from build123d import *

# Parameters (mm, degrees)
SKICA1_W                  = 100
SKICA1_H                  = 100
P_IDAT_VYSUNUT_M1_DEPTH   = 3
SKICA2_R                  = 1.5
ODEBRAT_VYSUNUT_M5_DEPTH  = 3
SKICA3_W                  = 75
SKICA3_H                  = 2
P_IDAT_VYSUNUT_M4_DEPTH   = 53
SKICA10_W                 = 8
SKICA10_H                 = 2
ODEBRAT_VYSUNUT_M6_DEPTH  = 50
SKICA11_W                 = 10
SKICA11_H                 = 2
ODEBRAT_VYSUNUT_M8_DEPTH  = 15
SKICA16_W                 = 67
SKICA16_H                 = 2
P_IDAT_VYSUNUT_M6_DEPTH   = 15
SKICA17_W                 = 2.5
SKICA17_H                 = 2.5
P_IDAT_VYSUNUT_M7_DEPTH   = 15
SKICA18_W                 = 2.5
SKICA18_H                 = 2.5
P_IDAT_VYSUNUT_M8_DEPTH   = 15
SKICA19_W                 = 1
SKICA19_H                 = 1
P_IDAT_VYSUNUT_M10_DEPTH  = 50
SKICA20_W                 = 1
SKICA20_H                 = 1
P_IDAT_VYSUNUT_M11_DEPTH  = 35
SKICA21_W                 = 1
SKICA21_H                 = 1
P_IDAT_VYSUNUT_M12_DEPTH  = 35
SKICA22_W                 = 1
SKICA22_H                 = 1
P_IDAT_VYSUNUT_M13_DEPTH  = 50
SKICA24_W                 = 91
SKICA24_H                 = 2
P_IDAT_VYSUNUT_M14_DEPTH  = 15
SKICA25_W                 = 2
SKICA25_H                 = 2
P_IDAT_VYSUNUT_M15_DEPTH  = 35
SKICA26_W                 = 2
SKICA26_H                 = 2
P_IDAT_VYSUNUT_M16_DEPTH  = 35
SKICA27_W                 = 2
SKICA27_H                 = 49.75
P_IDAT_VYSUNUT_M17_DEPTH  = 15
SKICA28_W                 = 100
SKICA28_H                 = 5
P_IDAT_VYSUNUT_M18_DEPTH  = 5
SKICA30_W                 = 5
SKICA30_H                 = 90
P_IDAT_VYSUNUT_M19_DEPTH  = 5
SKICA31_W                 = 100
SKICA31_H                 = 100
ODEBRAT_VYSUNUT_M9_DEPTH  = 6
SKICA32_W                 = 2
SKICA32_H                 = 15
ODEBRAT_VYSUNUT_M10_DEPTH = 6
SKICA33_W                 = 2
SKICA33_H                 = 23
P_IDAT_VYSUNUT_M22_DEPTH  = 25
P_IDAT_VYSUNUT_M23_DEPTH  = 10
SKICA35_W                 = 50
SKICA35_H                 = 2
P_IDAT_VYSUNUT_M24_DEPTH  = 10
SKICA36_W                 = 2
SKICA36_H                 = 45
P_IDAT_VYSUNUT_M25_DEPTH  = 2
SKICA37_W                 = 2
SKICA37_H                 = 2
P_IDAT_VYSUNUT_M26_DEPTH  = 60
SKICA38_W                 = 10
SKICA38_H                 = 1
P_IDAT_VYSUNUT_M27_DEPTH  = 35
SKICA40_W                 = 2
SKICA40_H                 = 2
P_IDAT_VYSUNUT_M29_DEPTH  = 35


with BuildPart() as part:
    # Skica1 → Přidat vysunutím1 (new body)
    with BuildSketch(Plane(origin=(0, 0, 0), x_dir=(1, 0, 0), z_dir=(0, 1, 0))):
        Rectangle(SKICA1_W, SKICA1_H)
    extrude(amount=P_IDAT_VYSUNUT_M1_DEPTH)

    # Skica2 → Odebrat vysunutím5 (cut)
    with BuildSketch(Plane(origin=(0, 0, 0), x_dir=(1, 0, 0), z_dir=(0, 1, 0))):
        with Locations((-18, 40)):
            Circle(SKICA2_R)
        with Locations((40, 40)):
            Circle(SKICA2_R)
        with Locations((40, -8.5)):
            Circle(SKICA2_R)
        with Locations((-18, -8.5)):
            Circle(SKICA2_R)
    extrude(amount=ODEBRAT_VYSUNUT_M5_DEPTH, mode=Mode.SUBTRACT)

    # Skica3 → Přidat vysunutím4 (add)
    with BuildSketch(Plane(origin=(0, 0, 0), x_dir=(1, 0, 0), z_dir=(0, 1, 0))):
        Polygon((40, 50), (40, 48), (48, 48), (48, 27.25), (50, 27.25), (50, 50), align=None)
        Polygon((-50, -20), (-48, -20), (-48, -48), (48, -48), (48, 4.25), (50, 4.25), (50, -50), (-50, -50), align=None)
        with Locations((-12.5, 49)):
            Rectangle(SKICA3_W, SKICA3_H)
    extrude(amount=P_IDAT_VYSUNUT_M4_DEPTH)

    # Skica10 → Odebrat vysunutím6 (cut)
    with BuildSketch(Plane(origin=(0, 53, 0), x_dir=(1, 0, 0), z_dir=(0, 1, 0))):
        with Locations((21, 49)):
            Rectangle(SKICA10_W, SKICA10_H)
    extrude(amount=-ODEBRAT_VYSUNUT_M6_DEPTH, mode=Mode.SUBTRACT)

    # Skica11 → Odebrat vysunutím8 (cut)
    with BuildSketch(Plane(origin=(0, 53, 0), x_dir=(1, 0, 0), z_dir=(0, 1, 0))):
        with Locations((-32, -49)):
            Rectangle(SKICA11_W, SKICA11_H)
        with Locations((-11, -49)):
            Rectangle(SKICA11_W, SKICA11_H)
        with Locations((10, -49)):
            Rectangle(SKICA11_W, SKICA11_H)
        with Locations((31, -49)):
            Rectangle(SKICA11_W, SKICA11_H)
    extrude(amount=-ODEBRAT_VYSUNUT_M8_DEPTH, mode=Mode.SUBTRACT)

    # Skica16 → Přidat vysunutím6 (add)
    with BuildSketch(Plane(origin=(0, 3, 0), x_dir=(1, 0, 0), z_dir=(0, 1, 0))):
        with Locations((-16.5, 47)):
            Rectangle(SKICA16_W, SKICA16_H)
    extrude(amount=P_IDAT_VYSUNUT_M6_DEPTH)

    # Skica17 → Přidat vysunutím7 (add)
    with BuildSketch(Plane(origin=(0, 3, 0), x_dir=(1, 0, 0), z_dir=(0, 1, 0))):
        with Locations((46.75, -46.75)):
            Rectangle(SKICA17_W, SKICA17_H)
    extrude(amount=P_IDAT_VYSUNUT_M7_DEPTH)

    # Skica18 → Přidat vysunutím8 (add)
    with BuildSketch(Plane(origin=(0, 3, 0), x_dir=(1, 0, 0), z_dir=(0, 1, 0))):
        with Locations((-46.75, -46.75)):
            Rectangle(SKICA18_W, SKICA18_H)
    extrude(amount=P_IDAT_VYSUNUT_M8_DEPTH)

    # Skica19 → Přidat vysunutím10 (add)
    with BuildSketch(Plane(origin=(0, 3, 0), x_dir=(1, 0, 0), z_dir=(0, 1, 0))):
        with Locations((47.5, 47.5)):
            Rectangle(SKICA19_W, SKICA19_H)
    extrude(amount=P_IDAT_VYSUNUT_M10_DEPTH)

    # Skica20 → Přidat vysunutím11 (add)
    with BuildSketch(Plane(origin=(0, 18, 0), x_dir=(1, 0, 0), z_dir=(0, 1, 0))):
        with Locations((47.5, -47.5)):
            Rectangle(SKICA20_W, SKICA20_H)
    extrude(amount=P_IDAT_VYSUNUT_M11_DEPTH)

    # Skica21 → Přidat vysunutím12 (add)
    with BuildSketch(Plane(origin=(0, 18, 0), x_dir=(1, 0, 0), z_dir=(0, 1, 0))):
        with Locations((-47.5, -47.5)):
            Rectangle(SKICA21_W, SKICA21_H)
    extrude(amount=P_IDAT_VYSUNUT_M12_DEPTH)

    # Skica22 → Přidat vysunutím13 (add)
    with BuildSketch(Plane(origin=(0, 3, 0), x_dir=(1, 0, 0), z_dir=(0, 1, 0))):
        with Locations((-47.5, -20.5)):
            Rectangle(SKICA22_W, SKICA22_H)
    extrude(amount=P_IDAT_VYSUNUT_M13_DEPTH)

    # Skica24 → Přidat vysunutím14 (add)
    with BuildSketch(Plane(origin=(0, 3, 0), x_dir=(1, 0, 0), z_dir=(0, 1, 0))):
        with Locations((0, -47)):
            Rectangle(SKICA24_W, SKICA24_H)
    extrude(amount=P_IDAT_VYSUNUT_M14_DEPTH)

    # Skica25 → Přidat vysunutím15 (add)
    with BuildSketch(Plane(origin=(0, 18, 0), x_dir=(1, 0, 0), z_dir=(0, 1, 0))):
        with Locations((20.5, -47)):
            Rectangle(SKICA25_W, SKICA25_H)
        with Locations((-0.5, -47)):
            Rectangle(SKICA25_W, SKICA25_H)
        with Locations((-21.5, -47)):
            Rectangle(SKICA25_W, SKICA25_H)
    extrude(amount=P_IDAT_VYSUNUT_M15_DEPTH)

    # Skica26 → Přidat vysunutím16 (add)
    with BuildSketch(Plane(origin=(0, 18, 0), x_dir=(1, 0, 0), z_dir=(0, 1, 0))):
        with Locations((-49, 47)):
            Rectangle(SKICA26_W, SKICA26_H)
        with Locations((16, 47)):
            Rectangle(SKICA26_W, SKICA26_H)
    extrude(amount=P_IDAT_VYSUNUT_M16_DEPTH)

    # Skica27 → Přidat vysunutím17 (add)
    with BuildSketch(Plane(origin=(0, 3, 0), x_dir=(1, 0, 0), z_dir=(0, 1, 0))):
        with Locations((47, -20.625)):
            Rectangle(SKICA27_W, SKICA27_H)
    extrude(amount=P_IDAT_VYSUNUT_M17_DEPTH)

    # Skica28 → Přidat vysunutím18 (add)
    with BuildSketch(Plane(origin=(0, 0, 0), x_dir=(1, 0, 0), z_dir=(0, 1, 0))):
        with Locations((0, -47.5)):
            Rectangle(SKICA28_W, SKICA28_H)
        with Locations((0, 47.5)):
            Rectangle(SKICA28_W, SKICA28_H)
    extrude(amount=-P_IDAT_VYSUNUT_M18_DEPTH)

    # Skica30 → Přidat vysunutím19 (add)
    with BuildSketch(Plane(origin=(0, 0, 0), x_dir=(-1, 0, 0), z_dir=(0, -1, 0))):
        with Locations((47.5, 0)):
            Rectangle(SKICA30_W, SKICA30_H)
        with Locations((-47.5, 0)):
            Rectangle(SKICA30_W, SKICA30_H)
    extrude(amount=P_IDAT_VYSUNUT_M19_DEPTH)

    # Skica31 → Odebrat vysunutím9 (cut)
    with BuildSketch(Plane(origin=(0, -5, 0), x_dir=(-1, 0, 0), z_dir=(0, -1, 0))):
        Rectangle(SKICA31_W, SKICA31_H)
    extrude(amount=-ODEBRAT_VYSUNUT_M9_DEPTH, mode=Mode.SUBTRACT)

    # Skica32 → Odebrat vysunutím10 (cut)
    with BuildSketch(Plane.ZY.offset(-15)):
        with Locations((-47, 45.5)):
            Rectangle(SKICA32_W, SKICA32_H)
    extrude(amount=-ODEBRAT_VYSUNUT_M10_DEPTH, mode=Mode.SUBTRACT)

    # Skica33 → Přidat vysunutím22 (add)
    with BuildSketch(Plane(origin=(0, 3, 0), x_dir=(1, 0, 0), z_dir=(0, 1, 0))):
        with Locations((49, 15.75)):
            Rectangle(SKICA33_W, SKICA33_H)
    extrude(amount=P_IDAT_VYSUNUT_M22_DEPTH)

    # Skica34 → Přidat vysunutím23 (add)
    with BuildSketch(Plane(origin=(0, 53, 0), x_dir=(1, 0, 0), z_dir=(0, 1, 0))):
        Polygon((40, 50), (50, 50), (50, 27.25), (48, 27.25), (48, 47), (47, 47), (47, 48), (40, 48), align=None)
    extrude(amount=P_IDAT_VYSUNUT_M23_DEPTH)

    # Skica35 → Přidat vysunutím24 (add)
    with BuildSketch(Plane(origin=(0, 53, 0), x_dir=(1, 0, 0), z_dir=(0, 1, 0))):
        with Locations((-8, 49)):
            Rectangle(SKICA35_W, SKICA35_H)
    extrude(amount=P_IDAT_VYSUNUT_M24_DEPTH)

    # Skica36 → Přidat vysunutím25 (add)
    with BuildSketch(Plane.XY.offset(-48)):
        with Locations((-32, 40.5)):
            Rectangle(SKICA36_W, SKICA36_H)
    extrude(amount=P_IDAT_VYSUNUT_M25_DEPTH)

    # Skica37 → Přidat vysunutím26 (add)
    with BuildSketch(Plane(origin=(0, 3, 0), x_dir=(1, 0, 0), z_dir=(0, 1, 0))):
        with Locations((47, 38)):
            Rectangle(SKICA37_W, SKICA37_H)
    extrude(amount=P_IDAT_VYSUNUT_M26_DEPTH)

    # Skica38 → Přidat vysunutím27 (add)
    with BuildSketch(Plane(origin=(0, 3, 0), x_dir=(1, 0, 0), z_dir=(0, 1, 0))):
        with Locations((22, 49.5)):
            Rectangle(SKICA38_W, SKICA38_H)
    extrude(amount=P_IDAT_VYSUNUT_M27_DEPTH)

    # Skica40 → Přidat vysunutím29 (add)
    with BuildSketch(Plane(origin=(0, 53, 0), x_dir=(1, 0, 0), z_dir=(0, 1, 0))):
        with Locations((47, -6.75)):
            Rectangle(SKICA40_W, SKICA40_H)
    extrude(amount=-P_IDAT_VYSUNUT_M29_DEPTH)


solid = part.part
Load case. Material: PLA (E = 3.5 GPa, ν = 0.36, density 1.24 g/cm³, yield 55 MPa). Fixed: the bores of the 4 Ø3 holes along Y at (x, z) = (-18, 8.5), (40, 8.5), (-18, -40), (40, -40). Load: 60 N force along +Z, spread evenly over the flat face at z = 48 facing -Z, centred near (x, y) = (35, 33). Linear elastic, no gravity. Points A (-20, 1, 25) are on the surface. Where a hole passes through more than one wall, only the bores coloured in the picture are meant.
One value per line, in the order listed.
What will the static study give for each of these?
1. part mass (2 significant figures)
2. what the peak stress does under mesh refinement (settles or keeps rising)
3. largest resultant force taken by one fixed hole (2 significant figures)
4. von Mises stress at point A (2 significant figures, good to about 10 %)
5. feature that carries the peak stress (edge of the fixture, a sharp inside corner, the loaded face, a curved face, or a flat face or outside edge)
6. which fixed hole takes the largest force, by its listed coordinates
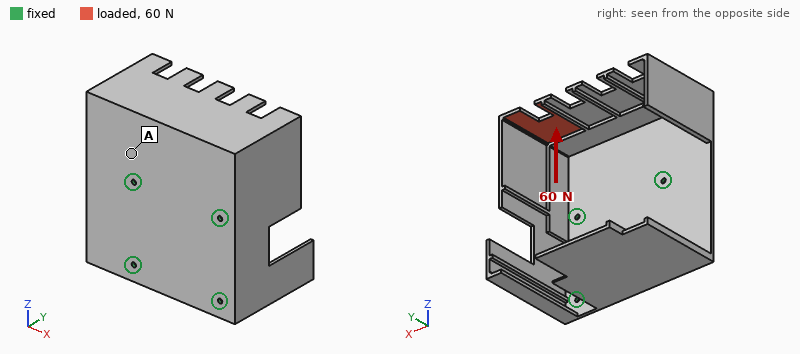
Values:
71 g
keeps rising
53 N
1.3 MPa
edge of the fixture
(40, -40)
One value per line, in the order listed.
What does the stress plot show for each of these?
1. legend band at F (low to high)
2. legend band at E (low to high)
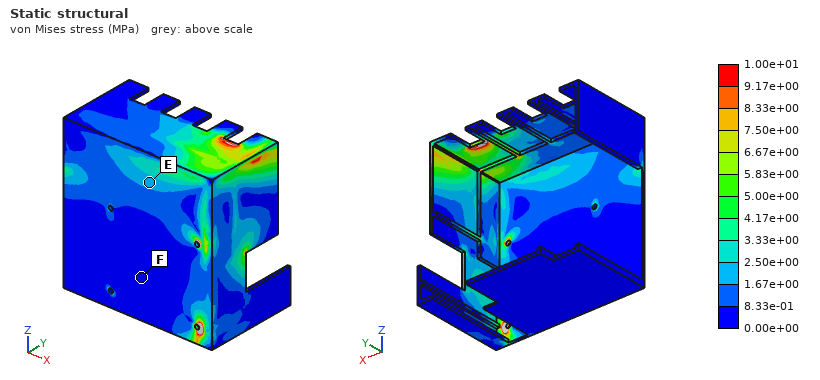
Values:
0.00e+00 to 8.33e-01 MPa
1.67e+00 to 2.50e+00 MPa
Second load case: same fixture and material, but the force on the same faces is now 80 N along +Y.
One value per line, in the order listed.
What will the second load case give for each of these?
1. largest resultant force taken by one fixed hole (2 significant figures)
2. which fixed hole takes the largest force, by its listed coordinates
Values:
140 N
(40, 8.5)
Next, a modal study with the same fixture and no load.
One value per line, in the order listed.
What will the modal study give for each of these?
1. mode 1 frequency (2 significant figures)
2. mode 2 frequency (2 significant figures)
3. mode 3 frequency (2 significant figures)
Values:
130 Hz
170 Hz
220 Hz
